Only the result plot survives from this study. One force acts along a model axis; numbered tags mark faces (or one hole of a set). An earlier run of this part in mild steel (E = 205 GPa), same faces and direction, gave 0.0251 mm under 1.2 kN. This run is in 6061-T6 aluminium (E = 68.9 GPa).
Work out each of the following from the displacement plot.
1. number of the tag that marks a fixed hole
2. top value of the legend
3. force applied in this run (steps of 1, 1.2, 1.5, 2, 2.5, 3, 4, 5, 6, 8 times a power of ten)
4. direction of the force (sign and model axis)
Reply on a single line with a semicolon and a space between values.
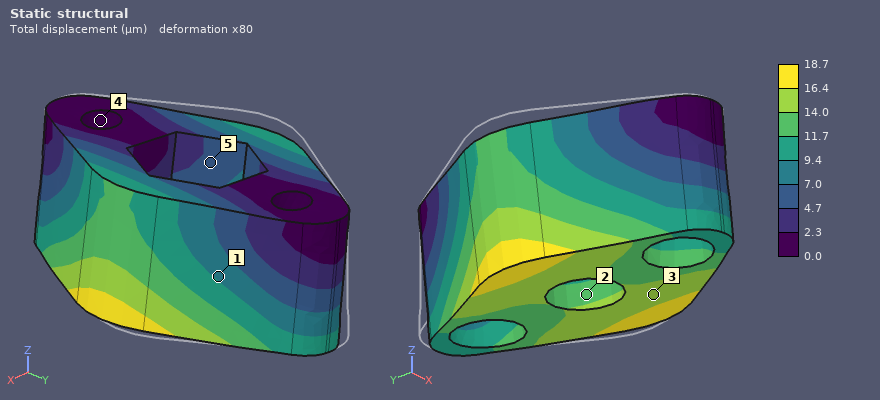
4; 18.7 µm; 300 N; +X
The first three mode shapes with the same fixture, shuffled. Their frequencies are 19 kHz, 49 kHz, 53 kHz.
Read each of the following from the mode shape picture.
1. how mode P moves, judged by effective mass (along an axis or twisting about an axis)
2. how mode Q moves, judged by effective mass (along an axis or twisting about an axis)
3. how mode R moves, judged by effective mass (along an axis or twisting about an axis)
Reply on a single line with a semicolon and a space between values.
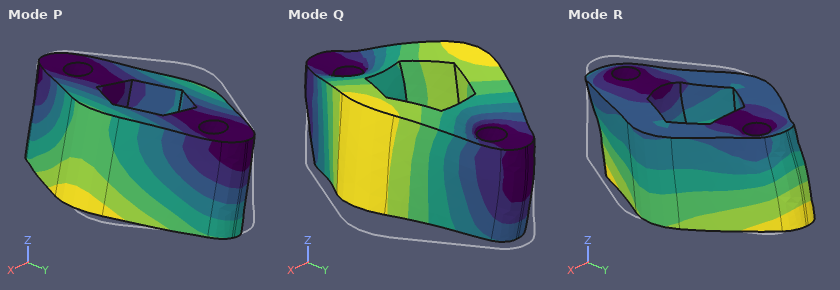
along X; along Z; along Y
